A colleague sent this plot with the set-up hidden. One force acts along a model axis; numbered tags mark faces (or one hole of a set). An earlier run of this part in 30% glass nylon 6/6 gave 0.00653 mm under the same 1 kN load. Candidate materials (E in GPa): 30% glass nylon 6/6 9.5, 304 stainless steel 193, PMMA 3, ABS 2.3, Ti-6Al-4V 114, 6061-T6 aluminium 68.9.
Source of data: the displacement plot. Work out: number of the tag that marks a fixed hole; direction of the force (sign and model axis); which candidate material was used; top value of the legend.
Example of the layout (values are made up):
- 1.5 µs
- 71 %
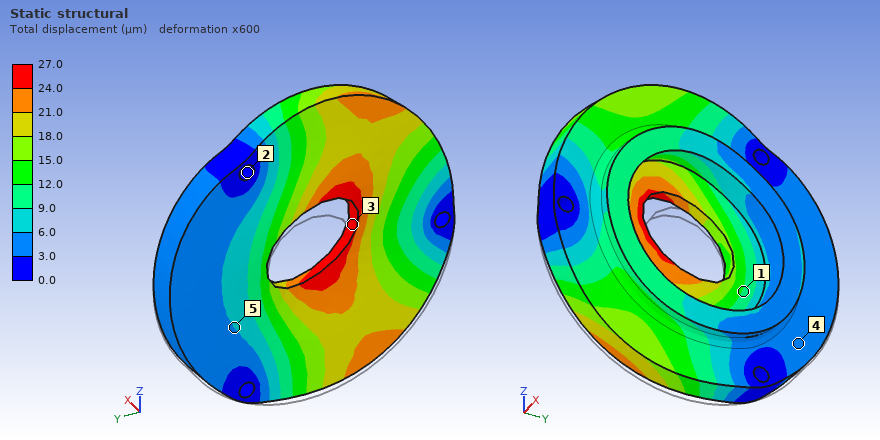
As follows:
- 2
- +Z
- ABS
- 27.0 µm
